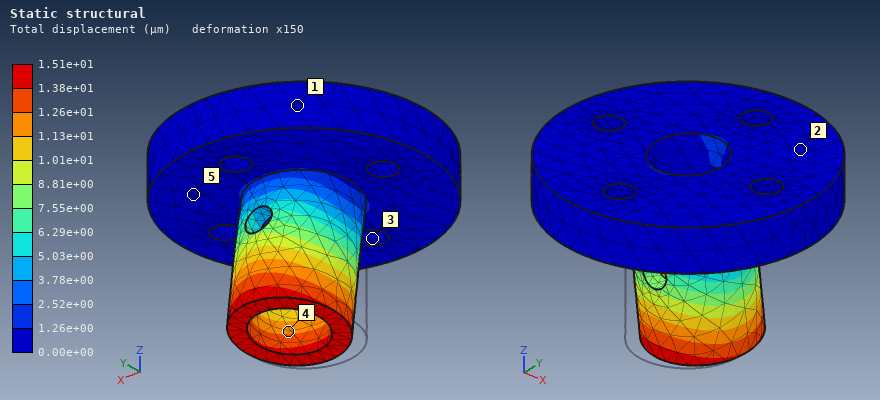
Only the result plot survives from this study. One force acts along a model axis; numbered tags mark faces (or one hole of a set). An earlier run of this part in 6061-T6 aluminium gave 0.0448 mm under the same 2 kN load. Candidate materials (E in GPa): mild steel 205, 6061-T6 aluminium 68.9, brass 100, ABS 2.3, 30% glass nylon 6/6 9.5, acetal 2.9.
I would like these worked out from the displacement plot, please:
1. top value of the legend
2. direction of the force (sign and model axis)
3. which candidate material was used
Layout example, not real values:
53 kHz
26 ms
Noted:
1.51e+01 µm
+Y
mild steel
